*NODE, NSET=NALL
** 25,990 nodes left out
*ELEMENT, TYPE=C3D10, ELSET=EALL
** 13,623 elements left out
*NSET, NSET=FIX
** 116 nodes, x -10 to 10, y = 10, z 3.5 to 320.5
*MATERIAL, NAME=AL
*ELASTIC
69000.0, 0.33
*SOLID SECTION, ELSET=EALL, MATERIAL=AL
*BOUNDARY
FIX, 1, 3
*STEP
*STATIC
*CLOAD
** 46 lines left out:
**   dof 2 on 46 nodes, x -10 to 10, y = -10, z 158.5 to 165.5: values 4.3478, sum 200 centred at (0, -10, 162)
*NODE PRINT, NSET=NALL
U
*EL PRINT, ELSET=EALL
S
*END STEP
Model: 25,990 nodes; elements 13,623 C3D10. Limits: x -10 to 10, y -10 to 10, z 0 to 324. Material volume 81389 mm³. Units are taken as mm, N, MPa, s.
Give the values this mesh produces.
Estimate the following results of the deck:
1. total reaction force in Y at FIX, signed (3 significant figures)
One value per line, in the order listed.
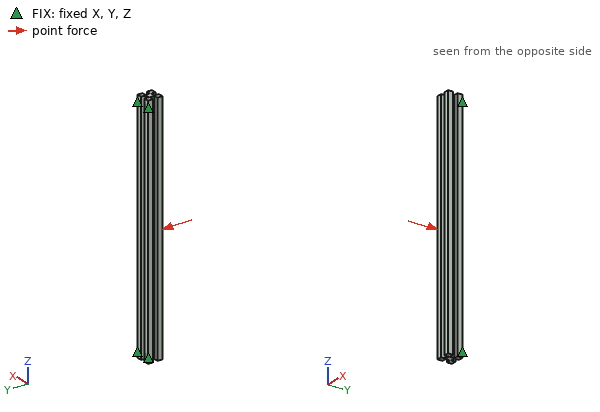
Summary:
-200 N
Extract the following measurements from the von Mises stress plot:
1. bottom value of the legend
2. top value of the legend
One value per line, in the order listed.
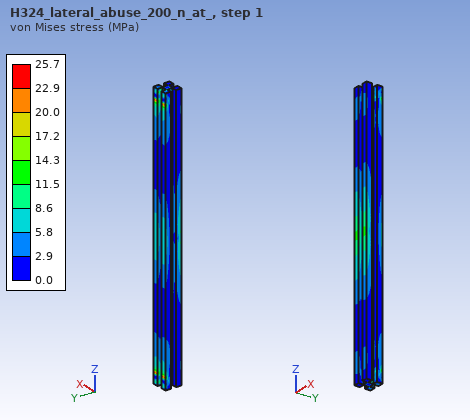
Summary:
0.0 MPa
25.7 MPa
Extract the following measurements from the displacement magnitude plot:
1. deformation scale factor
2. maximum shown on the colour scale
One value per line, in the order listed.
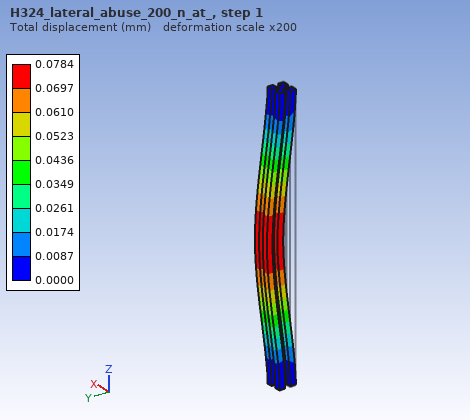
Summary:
200
0.0784 mm
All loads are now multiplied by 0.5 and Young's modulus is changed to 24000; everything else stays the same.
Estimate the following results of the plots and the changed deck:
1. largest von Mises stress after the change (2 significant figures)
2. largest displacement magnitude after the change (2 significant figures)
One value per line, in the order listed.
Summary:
13 MPa
0.11 mm
